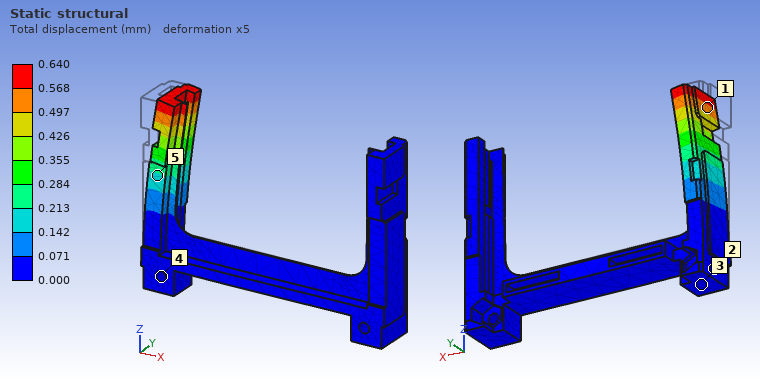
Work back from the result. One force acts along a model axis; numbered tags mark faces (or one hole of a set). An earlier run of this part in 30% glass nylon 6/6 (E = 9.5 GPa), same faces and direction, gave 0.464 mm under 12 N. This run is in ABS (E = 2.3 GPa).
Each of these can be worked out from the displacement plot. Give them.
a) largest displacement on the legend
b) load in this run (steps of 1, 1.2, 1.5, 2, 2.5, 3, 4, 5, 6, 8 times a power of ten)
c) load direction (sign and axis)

0.640 mm
4 N
+X
